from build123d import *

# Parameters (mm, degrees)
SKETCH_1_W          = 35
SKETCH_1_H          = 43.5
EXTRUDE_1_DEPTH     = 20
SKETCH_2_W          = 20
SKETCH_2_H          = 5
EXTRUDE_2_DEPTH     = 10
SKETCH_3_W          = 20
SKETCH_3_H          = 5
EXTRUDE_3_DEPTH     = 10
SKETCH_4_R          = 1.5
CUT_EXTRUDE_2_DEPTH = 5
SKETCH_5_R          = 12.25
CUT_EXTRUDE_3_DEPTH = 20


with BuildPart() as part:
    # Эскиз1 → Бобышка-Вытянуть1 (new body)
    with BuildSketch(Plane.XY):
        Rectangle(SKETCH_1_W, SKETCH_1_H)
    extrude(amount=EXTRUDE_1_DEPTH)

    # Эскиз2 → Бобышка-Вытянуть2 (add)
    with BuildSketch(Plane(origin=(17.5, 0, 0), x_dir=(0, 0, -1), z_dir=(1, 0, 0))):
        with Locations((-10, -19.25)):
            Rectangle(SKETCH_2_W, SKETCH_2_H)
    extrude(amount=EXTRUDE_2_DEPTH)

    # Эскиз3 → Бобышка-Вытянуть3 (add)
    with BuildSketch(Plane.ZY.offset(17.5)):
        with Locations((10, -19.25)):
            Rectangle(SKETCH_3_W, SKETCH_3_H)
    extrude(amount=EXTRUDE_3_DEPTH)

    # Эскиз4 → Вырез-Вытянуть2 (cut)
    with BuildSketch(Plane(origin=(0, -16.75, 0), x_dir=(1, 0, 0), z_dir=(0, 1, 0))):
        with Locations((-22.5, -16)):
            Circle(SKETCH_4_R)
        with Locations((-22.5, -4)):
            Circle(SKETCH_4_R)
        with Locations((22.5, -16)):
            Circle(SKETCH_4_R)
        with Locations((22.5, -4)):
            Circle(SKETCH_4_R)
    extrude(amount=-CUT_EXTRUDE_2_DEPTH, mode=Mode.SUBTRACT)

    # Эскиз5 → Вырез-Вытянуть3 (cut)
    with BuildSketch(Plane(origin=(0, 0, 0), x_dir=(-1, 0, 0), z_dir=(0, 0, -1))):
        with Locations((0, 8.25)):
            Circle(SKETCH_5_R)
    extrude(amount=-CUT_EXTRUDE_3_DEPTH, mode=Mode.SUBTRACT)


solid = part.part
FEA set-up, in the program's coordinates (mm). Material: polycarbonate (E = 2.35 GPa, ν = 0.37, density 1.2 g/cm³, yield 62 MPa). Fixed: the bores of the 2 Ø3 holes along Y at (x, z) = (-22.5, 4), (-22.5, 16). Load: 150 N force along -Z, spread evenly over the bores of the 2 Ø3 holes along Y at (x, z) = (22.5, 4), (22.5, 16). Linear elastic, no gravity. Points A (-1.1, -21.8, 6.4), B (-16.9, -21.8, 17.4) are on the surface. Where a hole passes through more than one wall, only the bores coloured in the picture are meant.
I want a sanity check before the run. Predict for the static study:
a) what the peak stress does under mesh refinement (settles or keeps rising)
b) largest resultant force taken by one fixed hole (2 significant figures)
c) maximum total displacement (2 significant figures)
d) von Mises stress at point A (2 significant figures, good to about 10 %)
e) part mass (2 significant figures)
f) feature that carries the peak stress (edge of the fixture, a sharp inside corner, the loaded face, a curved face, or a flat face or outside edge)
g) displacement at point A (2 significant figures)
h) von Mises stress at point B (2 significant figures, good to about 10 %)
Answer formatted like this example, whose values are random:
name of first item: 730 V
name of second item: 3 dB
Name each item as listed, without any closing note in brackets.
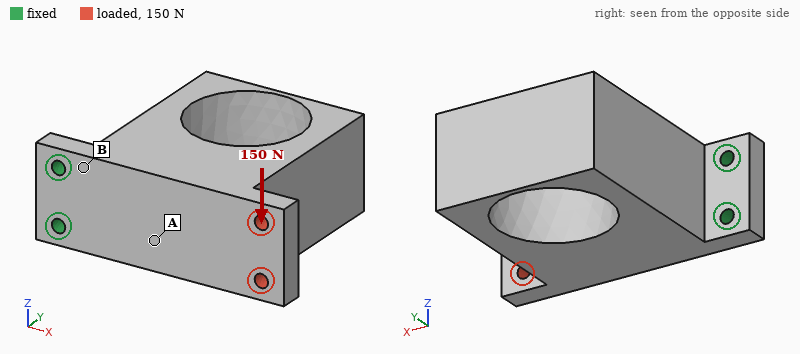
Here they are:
what the peak stress does under mesh refinement: keeps rising
largest resultant force taken by one fixed hole: 500 N
maximum total displacement: 0.60 mm
von Mises stress at point A: 3.2 MPa
part mass: 27 g
feature that carries the peak stress: edge of the fixture
displacement at point A: 0.20 mm
von Mises stress at point B: 11 MPa
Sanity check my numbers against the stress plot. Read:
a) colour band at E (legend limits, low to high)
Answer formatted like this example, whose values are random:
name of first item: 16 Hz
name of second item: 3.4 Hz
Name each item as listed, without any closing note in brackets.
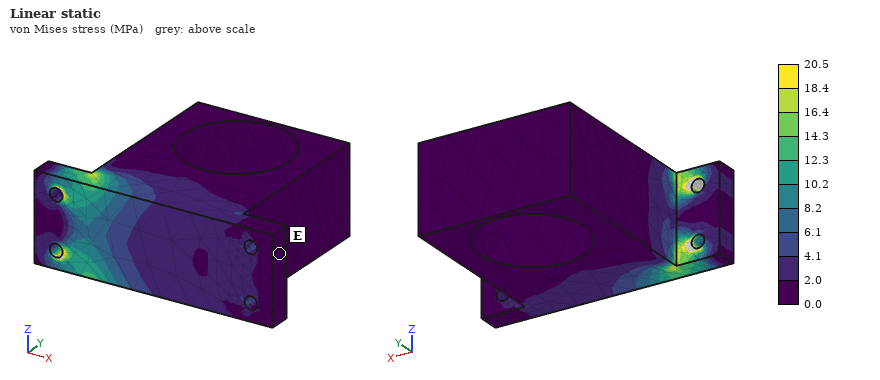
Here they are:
colour band at E: 0.0 to 2.0 MPa
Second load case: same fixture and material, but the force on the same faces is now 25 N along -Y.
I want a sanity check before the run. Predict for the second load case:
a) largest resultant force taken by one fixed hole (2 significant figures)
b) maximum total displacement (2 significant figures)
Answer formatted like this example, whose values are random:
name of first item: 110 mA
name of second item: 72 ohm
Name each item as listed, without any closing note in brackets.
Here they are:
largest resultant force taken by one fixed hole: 13 N
maximum total displacement: 0.85 mm
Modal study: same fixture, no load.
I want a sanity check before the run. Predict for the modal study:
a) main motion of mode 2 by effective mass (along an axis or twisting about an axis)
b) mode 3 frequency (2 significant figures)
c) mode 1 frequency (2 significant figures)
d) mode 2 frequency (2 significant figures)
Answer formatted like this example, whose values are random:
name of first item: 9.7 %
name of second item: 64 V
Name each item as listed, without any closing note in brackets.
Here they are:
main motion of mode 2 by effective mass: along Z
mode 3 frequency: 1200 Hz
mode 1 frequency: 260 Hz
mode 2 frequency: 700 Hz
